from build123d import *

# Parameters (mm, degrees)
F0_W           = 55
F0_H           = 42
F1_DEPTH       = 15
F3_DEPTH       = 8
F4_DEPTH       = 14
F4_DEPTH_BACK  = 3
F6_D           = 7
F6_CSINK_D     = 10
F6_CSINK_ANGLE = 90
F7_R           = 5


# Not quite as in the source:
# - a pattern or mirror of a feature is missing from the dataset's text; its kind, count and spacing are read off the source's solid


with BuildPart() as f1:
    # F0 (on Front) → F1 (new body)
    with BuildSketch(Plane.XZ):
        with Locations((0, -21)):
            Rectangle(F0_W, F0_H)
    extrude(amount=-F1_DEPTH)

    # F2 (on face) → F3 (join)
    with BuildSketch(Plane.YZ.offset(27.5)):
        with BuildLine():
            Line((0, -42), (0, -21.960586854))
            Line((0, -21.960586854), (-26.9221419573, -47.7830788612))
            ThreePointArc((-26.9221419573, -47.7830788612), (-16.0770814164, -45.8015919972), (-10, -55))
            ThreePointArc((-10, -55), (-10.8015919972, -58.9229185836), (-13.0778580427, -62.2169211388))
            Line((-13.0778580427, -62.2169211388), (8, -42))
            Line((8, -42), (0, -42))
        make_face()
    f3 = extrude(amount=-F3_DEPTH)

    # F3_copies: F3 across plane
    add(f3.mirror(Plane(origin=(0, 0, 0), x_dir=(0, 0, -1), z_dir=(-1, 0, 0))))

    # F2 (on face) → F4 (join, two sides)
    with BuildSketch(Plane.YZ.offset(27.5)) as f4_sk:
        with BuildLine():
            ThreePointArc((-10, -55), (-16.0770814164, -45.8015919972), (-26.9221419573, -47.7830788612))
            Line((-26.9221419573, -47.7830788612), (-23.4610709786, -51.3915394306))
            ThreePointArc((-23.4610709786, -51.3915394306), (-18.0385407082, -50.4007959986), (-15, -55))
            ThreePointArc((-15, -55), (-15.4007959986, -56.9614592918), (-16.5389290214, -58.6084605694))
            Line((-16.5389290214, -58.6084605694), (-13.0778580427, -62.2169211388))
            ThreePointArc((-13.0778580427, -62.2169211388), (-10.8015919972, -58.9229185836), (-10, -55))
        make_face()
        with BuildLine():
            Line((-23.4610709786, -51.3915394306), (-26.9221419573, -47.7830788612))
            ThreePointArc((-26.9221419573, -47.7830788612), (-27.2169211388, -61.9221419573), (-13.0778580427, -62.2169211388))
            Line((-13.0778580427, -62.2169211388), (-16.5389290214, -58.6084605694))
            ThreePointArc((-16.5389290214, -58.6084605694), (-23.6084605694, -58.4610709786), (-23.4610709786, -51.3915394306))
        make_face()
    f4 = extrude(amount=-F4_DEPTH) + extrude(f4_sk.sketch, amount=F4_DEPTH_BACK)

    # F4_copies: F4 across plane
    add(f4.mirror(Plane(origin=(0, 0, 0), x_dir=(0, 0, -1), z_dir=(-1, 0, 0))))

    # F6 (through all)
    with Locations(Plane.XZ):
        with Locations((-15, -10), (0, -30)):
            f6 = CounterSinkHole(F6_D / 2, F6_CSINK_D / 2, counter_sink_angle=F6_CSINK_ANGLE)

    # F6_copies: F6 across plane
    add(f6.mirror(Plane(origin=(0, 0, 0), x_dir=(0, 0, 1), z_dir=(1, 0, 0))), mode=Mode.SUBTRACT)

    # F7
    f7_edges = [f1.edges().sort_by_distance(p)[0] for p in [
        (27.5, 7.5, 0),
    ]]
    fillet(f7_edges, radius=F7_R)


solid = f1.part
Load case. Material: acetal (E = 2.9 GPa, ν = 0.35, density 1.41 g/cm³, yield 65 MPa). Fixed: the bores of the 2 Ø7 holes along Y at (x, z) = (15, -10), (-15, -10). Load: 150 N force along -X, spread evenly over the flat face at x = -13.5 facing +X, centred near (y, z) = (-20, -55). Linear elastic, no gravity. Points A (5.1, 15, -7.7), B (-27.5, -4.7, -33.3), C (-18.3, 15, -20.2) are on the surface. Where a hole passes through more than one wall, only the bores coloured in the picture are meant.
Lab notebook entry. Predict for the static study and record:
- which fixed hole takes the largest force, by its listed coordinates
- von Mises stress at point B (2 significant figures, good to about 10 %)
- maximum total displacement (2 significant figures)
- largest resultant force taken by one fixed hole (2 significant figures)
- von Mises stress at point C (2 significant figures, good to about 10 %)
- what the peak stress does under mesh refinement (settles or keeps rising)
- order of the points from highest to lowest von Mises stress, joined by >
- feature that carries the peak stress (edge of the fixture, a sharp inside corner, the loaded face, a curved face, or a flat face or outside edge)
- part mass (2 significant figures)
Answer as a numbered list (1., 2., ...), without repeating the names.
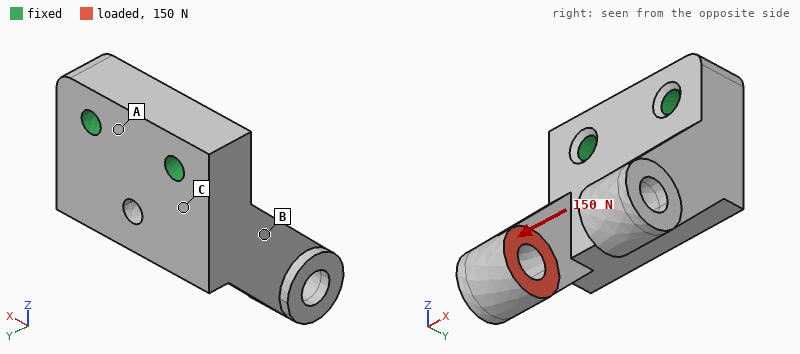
1. (15, -10)
2. 13 MPa
3. 1.1 mm
4. 240 N
5. 3.2 MPa
6. keeps rising
7. B > C > A
8. a sharp inside corner
9. 67 g
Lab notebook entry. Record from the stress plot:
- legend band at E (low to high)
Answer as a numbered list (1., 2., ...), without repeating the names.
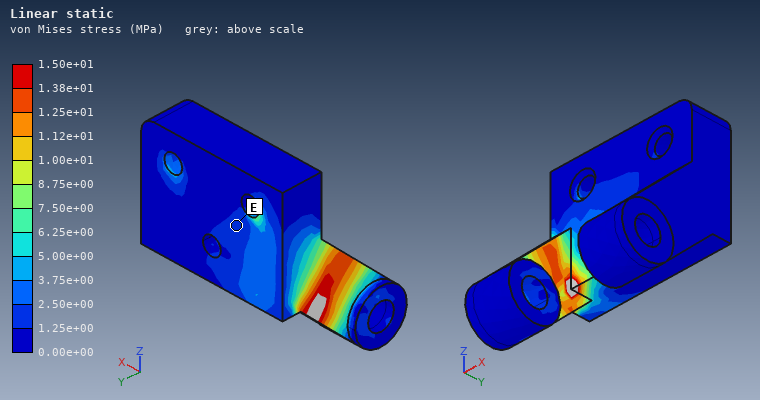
1. 1.25e+00 to 2.50e+00 MPa
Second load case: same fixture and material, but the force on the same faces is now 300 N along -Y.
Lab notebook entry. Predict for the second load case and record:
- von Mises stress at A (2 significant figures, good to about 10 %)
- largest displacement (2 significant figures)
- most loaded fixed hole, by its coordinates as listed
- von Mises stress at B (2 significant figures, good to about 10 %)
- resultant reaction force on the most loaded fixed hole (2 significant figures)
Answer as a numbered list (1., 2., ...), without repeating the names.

1. 2.1 MPa
2. 1.2 mm
3. (-15, -10)
4. 13 MPa
5. 250 N
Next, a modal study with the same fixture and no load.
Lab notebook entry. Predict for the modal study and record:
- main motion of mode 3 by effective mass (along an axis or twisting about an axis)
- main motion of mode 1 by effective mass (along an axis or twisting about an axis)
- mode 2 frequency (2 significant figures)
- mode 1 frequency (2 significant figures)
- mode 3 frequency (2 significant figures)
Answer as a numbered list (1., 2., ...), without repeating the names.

1. along Y
2. along X
3. 890 Hz
4. 850 Hz
5. 990 Hz
